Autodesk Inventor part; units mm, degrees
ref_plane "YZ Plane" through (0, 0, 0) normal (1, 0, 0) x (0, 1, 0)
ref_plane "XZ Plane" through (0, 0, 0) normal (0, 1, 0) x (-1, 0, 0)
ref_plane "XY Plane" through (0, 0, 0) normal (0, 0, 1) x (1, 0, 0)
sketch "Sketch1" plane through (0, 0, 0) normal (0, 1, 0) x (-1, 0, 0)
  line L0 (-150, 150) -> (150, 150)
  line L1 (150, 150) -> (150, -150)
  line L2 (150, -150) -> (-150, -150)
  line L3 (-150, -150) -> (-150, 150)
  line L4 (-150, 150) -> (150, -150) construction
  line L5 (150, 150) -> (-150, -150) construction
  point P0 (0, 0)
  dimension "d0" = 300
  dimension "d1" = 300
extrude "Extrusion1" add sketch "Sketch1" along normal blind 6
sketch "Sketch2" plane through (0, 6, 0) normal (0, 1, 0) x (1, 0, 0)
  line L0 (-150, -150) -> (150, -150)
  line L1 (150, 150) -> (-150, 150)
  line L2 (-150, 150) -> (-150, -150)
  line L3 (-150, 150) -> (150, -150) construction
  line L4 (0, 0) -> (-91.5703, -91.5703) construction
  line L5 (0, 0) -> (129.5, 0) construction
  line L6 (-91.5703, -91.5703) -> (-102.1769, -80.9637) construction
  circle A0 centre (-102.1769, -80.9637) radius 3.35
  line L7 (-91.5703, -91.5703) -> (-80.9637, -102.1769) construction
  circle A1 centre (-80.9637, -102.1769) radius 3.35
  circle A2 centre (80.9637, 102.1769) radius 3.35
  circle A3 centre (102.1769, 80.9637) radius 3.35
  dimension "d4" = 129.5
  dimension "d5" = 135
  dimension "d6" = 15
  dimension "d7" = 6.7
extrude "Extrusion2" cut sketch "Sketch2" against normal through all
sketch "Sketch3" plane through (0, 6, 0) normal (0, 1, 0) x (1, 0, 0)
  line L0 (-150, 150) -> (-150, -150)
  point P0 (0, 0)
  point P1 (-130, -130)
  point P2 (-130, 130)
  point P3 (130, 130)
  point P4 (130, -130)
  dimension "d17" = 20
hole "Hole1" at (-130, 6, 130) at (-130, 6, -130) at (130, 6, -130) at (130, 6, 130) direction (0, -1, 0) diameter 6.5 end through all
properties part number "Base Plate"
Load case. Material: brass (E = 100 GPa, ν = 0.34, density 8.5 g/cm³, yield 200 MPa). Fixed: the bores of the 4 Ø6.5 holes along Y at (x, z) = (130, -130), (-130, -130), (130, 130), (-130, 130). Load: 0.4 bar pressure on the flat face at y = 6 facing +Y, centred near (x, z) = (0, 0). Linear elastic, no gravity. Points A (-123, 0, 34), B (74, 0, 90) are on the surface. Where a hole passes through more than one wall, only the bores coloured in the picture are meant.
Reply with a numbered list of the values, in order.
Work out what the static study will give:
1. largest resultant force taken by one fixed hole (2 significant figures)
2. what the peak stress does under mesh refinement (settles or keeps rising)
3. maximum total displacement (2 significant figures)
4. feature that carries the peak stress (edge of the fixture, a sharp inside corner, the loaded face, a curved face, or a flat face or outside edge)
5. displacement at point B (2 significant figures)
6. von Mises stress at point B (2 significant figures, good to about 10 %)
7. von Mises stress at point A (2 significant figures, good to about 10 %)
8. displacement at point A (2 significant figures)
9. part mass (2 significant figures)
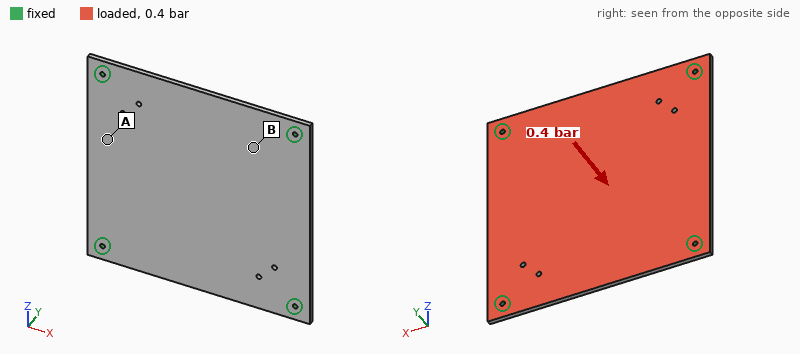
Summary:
1. 900 N
2. keeps rising
3. 0.79 mm
4. edge of the fixture
5. 0.39 mm
6. 11 MPa
7. 23 MPa
8. 0.42 mm
9. 4.6 kg
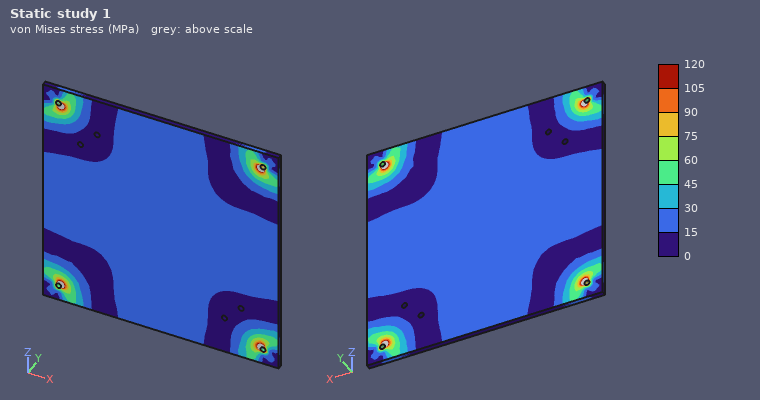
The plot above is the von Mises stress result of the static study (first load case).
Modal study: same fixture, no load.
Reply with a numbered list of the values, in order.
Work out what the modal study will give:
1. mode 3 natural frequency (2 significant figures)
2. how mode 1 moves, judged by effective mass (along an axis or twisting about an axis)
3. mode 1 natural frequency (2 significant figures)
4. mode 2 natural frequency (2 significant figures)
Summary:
1. 330 Hz
2. along Y
3. 190 Hz
4. 330 Hz
